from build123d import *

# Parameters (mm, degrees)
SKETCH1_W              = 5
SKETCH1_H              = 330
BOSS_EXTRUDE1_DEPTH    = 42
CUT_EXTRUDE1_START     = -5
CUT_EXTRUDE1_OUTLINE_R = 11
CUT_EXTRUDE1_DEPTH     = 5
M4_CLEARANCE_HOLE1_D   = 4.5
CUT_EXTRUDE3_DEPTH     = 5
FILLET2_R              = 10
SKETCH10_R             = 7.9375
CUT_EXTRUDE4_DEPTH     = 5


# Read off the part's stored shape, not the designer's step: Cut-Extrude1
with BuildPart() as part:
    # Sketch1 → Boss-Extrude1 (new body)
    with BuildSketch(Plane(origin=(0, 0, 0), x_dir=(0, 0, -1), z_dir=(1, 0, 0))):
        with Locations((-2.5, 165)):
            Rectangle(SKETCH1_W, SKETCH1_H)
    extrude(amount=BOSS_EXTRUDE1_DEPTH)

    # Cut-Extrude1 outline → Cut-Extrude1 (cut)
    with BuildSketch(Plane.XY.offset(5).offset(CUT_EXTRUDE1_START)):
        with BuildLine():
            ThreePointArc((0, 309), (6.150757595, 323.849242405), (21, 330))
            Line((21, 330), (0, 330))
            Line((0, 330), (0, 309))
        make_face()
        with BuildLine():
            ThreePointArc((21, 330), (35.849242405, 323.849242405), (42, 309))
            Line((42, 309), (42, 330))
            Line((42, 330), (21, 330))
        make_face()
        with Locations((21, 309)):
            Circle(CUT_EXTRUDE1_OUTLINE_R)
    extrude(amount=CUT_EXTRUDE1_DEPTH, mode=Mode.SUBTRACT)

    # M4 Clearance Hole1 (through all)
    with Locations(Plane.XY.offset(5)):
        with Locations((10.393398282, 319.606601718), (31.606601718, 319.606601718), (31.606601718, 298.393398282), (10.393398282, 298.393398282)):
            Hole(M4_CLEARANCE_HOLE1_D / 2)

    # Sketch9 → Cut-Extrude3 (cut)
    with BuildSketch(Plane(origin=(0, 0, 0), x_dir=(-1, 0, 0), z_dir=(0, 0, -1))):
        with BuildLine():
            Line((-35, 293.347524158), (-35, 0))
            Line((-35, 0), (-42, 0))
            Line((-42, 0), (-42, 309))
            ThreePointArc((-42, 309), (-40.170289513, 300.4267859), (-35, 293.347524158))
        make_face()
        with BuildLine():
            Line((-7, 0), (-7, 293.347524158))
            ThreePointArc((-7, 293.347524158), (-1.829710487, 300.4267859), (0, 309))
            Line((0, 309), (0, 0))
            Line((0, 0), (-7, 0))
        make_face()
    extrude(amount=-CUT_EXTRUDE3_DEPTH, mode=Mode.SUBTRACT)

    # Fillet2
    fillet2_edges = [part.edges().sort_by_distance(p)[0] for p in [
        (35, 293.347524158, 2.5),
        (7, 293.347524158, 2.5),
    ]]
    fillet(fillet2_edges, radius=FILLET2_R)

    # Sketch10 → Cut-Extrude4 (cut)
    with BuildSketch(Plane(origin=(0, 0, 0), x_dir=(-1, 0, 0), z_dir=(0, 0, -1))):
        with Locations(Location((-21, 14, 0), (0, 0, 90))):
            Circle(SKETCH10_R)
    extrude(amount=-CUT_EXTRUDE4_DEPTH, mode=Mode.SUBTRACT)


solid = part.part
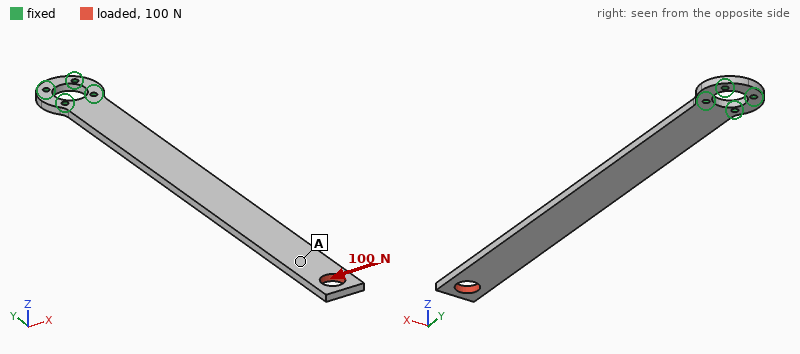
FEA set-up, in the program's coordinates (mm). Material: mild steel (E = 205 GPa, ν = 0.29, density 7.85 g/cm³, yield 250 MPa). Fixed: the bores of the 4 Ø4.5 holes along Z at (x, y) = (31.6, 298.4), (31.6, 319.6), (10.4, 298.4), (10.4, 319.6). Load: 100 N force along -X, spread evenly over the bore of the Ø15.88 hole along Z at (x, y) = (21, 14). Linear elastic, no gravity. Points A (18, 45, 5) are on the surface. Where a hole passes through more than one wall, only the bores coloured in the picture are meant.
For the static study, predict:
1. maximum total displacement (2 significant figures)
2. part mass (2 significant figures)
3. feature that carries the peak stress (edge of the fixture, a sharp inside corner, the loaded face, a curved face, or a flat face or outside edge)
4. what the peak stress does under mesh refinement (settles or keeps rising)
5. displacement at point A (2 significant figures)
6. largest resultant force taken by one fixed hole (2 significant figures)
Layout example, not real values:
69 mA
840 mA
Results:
0.44 mm
350 g
edge of the fixture
keeps rising
0.34 mm
1.2 kN
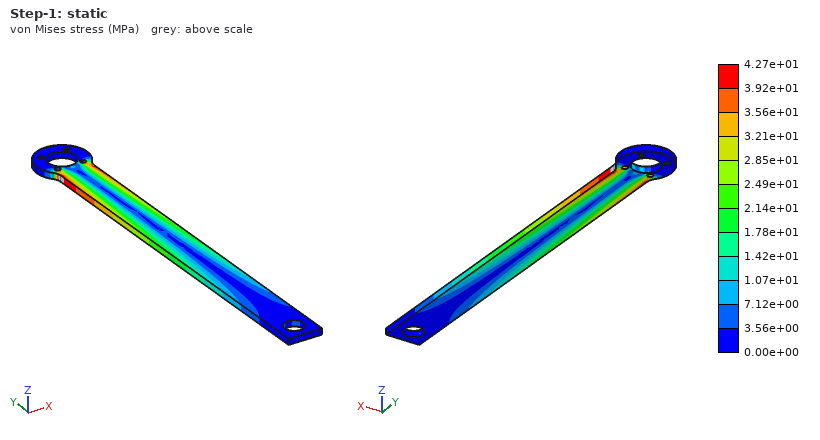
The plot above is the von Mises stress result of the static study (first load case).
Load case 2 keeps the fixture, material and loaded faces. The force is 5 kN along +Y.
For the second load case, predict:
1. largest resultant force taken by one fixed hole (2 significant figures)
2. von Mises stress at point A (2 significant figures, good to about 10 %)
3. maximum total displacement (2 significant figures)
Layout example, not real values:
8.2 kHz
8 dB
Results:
2.6 kN
34 MPa
58 µm
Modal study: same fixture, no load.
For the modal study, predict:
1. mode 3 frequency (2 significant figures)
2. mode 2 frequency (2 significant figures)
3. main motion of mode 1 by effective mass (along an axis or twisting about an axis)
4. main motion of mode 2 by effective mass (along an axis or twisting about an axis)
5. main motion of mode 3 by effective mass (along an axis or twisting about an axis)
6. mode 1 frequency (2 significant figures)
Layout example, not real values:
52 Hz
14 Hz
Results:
300 Hz
270 Hz
along Z
along X
along Z
48 Hz
